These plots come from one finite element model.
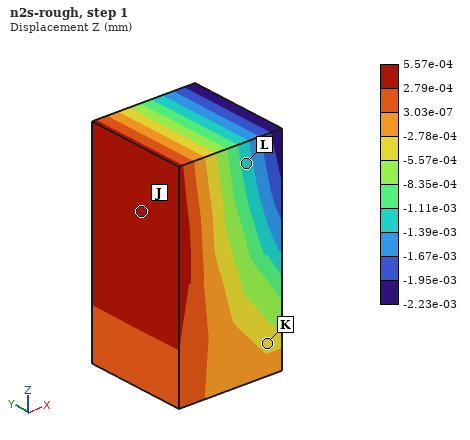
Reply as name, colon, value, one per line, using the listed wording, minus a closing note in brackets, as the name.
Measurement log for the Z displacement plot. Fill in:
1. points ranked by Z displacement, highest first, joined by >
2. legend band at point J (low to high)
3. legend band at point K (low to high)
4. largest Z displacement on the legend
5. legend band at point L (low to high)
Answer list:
points ranked by Z displacement, highest first, joined by >: J > K > L
legend band at point J: 2.79e-04 to 5.57e-04 mm
legend band at point K: -5.57e-04 to -2.78e-04 mm
largest Z displacement on the legend: 5.57e-04 mm
legend band at point L: -1.39e-03 to -1.11e-03 mm
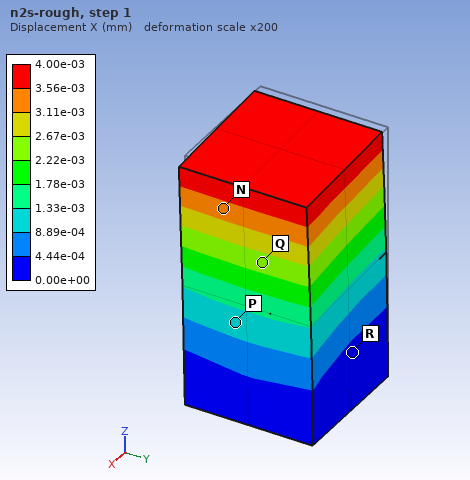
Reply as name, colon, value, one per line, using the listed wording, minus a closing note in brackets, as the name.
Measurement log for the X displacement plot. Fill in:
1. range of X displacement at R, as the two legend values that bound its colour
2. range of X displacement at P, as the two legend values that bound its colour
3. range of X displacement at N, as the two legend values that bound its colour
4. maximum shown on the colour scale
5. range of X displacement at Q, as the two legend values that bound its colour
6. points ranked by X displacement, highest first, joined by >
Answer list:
range of X displacement at R, as the two legend values that bound its colour: 0.00e+00 to 4.44e-04 mm
range of X displacement at P, as the two legend values that bound its colour: 8.89e-04 to 1.33e-03 mm
range of X displacement at N, as the two legend values that bound its colour: 3.11e-03 to 3.56e-03 mm
maximum shown on the colour scale: 4.00e-03 mm
range of X displacement at Q, as the two legend values that bound its colour: 2.22e-03 to 2.67e-03 mm
points ranked by X displacement, highest first, joined by >: N > Q > P > R
